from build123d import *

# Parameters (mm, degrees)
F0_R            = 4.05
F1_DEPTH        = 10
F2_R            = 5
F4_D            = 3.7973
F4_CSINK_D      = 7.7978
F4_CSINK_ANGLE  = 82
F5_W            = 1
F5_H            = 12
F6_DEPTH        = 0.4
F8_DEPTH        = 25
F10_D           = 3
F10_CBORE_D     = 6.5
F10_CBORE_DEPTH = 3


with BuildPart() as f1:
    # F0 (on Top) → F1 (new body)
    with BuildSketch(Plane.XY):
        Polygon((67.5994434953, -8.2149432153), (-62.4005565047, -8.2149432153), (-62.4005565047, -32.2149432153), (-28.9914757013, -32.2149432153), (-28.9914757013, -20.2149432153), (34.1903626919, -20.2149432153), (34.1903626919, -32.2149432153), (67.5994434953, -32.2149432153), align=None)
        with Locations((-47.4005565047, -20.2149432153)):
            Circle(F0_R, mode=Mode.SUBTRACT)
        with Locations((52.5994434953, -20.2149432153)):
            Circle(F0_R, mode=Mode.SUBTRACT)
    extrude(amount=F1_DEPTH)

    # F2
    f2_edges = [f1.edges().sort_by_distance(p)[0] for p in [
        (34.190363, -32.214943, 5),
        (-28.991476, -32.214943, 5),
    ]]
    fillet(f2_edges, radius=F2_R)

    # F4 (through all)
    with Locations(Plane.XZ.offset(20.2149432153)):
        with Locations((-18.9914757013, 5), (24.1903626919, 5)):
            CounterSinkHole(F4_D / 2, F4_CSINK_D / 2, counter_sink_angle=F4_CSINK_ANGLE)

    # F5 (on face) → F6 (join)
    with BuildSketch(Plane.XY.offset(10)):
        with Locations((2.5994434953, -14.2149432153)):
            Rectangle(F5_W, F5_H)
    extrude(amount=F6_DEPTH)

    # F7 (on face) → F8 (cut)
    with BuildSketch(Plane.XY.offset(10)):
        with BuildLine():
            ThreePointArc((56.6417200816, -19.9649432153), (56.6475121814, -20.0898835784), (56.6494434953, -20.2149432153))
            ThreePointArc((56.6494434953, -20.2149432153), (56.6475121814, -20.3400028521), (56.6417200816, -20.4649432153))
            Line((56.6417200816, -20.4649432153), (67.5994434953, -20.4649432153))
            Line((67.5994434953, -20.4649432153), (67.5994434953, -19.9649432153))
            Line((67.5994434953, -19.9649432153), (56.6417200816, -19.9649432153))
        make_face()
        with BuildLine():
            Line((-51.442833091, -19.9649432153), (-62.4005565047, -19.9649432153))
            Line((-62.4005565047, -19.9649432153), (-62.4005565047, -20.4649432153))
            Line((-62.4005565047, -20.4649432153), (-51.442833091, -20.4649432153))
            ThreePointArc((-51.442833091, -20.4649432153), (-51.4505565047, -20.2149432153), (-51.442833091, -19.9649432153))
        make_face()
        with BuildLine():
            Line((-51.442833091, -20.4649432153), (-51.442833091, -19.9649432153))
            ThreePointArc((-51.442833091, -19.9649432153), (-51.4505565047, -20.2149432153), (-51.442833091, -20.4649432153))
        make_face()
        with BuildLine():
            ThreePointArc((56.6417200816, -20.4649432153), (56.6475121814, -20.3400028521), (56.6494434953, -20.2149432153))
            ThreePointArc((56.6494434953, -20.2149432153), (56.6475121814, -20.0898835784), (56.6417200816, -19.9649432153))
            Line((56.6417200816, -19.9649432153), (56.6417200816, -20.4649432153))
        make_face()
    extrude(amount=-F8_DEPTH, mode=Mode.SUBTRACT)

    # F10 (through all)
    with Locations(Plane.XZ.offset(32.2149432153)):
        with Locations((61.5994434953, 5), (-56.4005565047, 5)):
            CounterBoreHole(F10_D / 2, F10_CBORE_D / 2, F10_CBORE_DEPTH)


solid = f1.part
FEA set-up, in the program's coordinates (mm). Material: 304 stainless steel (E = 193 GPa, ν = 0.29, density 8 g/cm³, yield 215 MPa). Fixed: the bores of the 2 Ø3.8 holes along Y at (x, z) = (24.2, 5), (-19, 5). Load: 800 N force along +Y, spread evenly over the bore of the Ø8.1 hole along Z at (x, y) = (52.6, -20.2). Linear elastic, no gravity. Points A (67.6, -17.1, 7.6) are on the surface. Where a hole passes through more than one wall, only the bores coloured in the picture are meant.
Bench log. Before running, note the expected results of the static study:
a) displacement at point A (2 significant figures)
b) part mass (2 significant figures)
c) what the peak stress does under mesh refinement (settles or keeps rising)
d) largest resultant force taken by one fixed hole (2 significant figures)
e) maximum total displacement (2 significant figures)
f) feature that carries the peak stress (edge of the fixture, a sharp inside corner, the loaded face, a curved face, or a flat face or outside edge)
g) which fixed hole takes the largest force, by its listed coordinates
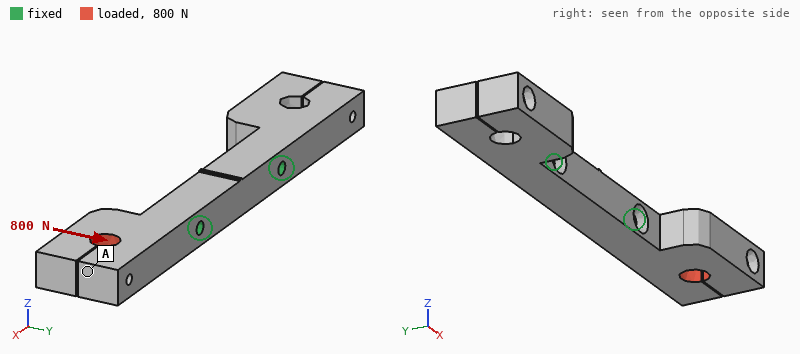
43 µm
170 g
keeps rising
870 N
49 µm
edge of the fixture
(24.2, 5)
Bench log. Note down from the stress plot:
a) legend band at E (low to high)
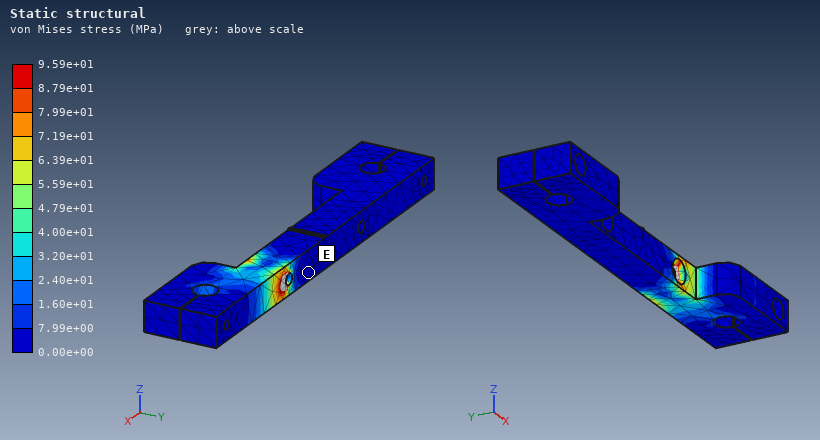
0.00e+00 to 7.99e+00 MPa
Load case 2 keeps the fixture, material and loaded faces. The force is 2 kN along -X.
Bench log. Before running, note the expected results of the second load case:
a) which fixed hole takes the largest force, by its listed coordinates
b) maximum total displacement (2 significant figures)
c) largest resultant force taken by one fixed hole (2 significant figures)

(24.2, 5)
33 µm
1.9 kN
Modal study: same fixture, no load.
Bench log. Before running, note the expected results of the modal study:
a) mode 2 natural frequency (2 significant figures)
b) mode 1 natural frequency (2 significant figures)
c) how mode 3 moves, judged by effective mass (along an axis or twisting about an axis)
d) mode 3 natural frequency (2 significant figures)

2800 Hz
2700 Hz
along Y
3400 Hz
